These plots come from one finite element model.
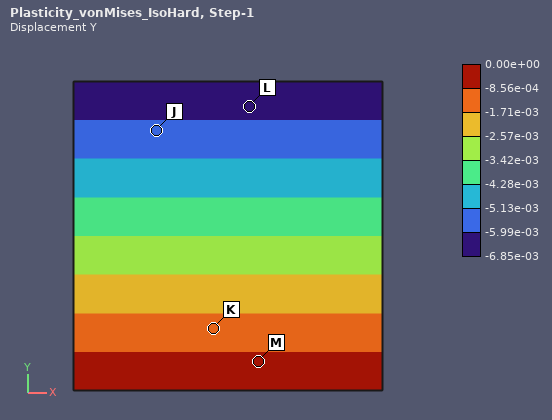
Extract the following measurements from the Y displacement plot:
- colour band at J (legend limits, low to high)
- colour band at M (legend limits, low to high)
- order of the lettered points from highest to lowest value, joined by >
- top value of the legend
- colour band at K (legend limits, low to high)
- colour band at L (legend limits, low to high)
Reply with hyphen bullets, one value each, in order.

- -5.99e-03 to -5.13e-03
- -8.56e-04 to 0.00e+00
- M > K > J > L
- 0.00e+00
- -1.71e-03 to -8.56e-04
- -6.85e-03 to -5.99e-03
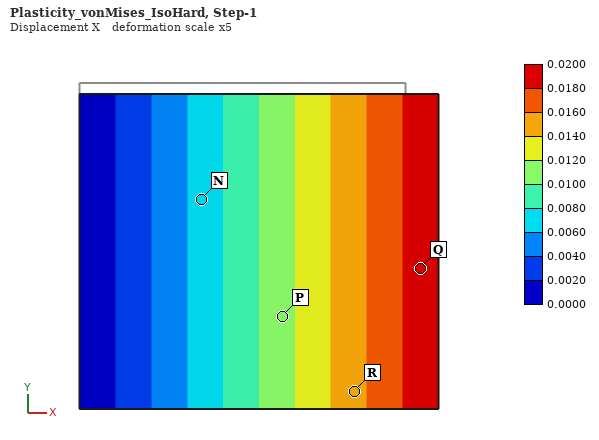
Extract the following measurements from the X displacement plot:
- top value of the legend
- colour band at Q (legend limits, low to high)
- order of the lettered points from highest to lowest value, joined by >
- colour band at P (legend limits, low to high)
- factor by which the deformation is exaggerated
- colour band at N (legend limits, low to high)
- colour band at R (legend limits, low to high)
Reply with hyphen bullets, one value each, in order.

- 0.0200
- 0.0180 to 0.0200
- Q > R > P > N
- 0.0100 to 0.0120
- 5
- 0.0060 to 0.0080
- 0.0140 to 0.0160
